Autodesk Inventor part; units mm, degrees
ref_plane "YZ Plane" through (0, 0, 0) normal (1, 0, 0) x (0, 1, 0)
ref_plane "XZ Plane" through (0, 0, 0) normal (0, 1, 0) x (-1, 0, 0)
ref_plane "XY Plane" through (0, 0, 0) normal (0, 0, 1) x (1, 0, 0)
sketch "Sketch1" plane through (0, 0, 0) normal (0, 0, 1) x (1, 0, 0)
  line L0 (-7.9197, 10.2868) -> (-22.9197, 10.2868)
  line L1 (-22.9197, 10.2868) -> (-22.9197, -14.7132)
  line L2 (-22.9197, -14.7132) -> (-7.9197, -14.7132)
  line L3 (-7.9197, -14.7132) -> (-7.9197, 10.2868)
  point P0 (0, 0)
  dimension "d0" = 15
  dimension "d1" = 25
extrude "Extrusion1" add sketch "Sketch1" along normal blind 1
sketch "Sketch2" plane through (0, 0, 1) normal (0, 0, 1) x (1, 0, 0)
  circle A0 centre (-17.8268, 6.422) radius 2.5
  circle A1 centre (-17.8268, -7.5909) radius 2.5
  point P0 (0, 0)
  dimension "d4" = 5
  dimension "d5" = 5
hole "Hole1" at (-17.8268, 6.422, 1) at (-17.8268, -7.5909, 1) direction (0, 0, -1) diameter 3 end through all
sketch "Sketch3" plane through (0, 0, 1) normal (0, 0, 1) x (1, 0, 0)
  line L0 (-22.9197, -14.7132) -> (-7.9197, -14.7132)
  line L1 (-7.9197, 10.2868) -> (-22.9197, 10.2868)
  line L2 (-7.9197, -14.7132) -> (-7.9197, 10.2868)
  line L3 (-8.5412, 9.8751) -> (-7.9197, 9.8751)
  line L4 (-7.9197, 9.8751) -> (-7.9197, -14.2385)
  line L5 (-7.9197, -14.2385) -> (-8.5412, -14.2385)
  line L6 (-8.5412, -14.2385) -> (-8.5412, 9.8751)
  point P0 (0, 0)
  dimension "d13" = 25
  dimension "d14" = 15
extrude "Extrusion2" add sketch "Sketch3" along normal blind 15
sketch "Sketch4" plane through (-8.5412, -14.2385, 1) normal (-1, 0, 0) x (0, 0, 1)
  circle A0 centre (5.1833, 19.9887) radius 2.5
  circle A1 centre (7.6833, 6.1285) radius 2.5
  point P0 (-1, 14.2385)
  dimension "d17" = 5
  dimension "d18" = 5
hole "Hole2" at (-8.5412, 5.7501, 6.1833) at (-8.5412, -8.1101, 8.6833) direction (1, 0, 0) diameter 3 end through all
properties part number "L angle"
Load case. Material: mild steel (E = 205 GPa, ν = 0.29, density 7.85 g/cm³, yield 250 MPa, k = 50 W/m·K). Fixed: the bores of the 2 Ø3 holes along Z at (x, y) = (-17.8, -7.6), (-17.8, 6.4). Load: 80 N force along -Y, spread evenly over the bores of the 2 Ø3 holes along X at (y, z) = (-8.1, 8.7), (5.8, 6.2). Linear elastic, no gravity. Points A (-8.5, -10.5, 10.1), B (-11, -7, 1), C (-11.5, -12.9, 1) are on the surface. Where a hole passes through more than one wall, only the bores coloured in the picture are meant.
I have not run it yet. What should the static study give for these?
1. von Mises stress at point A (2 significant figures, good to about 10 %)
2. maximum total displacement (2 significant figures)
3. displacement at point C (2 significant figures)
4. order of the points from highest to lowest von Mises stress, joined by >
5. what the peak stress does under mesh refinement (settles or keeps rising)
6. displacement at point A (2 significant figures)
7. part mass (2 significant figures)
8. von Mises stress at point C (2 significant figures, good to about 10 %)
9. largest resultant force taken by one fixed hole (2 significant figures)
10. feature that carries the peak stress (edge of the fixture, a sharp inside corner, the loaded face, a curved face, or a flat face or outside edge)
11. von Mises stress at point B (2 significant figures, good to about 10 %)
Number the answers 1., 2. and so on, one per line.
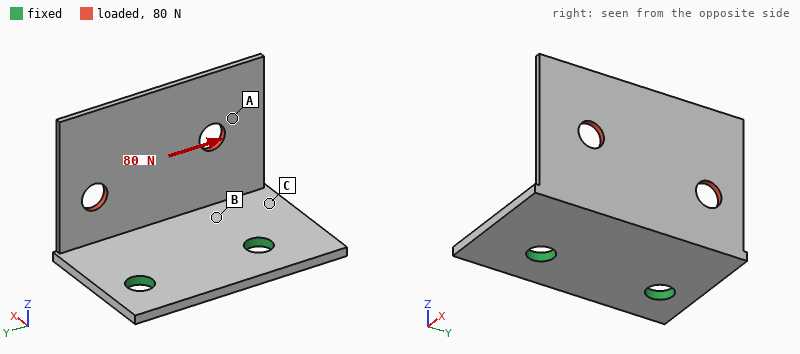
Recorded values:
1. 14 MPa
2. 70 µm
3. 20 µm
4. B > C > A
5. keeps rising
6. 45 µm
7. 4.5 g
8. 40 MPa
9. 70 N
10. edge of the fixture
11. 62 MPa
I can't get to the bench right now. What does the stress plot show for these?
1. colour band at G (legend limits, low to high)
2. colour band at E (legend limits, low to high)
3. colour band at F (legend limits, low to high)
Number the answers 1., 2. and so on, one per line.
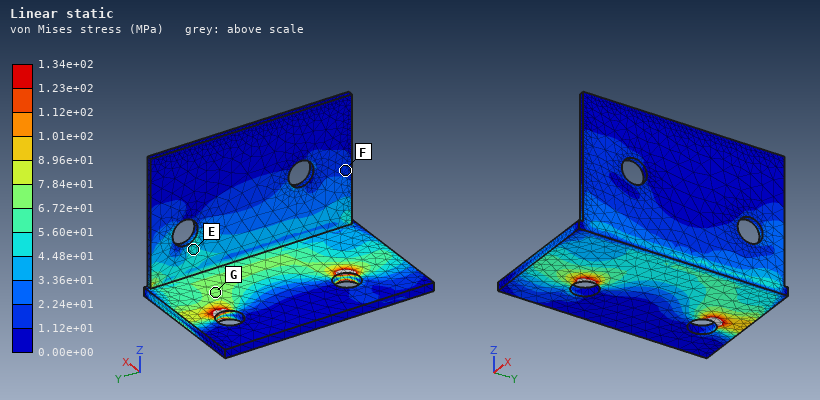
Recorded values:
1. 6.72e+01 to 7.84e+01 MPa
2. 4.48e+01 to 5.60e+01 MPa
3. 1.12e+01 to 2.24e+01 MPa
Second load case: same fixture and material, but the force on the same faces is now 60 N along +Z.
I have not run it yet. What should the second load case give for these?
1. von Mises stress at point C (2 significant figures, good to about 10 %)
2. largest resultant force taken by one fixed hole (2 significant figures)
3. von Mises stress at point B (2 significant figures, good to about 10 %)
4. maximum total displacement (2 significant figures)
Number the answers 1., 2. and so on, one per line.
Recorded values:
1. 42 MPa
2. 32 N
3. 33 MPa
4. 94 µm
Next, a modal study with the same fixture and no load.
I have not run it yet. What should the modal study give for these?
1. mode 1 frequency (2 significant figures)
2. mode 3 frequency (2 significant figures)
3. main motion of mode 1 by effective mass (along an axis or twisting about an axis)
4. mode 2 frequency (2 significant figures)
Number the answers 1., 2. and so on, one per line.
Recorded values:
1. 1800 Hz
2. 4700 Hz
3. along X
4. 3400 Hz
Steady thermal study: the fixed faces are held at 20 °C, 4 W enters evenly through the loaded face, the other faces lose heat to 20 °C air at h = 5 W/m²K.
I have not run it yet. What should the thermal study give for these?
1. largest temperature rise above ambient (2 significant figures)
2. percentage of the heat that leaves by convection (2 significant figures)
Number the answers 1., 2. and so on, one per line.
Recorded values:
1. 77 K
2. 6.4 %
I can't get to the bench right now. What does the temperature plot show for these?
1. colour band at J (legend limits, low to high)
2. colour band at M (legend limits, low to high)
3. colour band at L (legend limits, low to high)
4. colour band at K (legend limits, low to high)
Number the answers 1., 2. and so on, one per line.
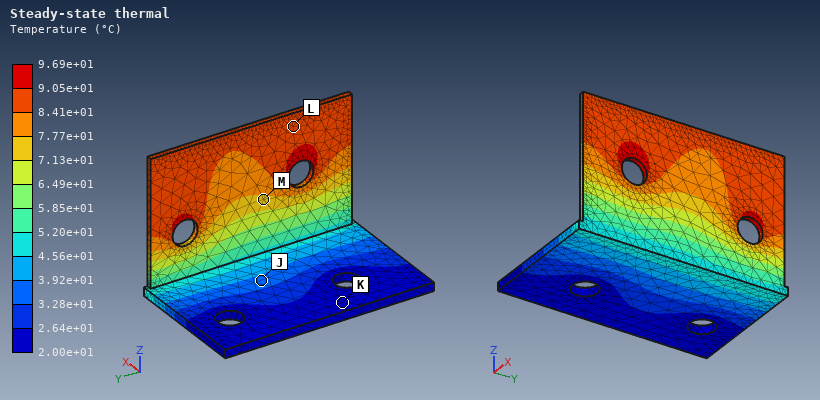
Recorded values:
1. 3.28e+01 to 3.92e+01 °C
2. 7.13e+01 to 7.77e+01 °C
3. 8.41e+01 to 9.05e+01 °C
4. 2.00e+01 to 2.64e+01 °C
